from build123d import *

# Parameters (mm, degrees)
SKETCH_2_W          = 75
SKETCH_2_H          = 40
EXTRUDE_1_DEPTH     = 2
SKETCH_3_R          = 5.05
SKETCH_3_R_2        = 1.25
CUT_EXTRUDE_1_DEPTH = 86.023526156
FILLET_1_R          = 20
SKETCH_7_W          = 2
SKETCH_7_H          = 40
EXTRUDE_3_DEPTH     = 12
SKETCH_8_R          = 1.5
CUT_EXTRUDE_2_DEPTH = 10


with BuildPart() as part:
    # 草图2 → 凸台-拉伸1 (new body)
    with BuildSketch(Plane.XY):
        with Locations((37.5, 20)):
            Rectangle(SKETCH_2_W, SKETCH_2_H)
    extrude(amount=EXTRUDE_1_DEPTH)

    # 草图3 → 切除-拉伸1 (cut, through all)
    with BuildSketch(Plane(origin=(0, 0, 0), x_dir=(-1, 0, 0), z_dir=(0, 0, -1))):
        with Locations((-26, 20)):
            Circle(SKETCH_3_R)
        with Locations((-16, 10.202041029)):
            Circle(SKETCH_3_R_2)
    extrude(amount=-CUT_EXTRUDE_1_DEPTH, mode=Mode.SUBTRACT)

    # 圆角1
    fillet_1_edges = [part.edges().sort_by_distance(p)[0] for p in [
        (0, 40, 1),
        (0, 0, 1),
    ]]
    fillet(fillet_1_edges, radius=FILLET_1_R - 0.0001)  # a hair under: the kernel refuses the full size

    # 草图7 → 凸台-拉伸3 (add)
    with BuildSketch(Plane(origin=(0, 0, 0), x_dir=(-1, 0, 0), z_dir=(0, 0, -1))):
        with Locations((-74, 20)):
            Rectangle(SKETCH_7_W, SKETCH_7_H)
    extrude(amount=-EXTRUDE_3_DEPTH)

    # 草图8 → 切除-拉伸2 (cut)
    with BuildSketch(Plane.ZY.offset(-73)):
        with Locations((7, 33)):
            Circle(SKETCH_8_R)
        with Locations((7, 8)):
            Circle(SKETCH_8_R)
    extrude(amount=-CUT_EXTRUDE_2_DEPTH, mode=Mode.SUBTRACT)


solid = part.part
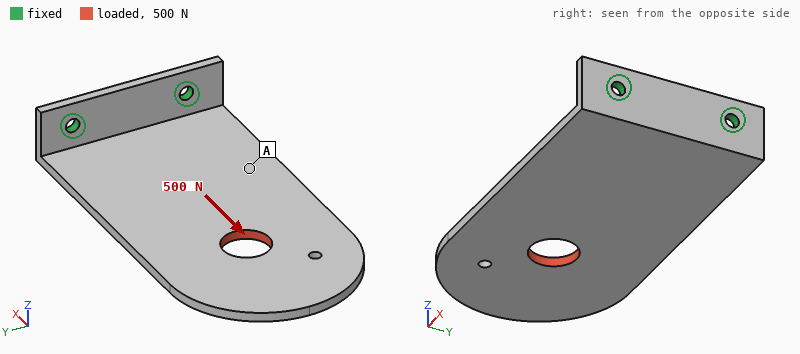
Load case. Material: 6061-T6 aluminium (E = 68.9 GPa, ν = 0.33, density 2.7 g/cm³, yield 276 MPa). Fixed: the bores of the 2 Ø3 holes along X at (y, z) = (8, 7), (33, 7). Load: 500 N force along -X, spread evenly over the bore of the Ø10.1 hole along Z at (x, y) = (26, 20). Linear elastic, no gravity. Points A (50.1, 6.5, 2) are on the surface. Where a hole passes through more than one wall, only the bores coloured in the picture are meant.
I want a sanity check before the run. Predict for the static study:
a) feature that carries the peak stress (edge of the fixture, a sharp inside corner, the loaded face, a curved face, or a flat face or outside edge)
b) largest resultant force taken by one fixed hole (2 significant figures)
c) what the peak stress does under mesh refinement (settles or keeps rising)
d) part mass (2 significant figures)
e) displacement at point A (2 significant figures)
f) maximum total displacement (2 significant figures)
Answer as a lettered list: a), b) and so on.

a) edge of the fixture
b) 260 N
c) keeps rising
d) 17 g
e) 0.13 mm
f) 0.40 mm
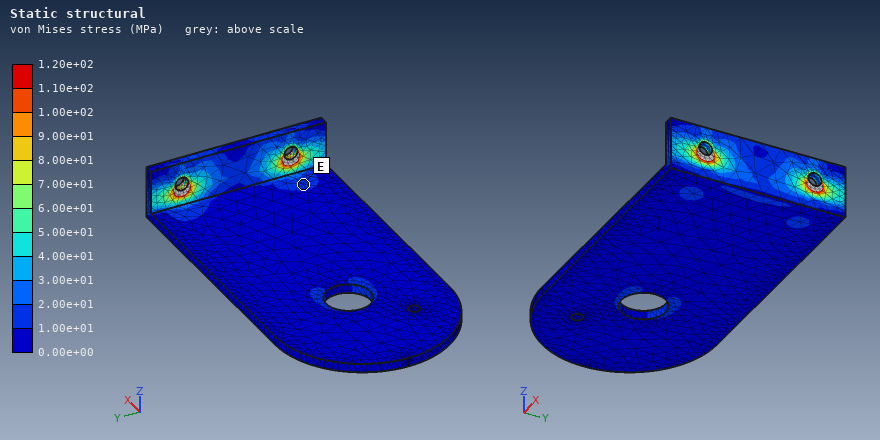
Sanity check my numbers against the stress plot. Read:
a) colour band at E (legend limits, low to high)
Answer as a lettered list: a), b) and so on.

a) 1.00e+01 to 2.00e+01 MPa
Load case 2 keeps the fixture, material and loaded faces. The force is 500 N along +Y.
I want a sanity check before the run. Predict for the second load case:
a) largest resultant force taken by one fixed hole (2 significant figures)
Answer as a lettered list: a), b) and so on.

a) 940 N
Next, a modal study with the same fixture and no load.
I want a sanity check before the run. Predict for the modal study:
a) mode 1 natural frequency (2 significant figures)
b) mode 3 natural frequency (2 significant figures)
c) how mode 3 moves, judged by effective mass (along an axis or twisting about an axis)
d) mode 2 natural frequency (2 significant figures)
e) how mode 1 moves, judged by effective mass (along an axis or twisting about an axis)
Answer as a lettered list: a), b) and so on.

a) 300 Hz
b) 1800 Hz
c) along Z
d) 1300 Hz
e) along Z
